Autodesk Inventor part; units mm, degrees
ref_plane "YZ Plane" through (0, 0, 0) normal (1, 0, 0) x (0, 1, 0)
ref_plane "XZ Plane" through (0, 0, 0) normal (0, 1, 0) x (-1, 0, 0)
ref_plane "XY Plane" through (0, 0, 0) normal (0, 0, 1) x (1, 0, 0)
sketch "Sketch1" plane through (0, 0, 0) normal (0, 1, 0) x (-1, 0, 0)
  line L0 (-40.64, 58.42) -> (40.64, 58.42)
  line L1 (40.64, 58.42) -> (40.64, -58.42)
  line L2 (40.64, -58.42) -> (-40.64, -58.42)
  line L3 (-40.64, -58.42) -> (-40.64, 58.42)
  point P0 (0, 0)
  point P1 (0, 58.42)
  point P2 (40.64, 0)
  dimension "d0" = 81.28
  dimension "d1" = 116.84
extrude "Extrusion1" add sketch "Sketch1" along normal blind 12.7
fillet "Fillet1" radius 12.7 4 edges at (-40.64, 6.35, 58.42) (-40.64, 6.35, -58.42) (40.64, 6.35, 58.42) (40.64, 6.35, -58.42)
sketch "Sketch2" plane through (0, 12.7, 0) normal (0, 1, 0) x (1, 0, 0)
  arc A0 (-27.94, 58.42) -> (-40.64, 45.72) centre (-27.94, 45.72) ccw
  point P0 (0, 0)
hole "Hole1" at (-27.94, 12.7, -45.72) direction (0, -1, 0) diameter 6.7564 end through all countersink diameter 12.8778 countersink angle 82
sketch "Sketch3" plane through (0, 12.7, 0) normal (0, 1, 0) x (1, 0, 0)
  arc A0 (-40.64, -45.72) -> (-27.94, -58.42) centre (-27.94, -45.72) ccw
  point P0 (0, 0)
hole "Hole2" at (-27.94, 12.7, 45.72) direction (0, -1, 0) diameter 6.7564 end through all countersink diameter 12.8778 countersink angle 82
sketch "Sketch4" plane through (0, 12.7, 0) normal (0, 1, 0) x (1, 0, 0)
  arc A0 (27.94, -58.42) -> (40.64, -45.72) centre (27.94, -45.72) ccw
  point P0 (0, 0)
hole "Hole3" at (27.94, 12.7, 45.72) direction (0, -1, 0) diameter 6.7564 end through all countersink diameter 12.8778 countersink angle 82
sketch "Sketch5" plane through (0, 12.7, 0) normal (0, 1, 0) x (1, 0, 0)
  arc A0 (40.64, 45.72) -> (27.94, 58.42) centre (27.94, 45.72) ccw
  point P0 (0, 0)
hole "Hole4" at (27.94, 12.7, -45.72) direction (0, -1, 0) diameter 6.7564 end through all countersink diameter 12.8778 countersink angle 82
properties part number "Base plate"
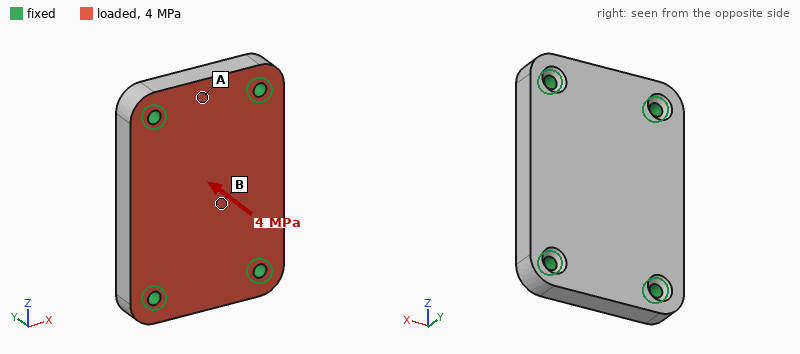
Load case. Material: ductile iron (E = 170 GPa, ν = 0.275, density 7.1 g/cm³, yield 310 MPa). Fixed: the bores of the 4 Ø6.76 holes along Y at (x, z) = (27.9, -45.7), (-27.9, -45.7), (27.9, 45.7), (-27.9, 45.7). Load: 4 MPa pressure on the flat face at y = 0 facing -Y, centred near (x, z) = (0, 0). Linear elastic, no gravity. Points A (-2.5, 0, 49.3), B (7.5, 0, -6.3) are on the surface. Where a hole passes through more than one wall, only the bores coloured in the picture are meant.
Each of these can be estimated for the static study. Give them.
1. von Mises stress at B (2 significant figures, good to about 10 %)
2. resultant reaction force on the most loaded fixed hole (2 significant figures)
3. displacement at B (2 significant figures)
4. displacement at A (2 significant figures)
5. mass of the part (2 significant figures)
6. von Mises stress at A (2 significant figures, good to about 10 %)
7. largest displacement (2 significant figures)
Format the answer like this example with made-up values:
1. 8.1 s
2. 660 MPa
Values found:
1. 50 MPa
2. 9.4 kN
3. 48 µm
4. 9.6 µm
5. 830 g
6. 30 MPa
7. 49 µm
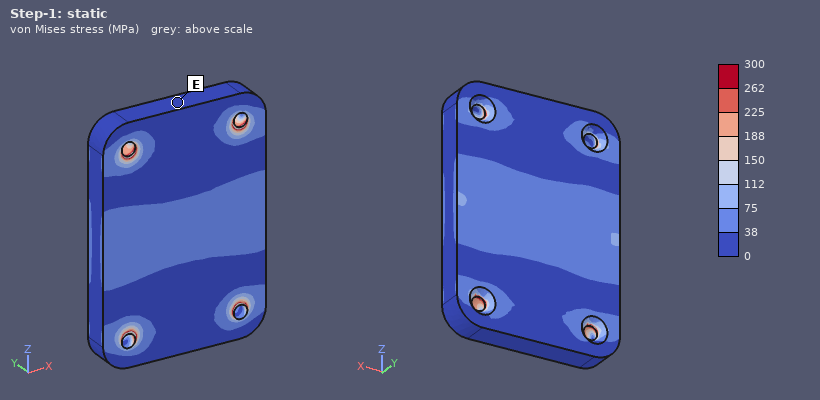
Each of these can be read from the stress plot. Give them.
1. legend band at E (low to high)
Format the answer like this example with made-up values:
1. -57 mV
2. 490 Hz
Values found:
1. 0 to 38 MPa
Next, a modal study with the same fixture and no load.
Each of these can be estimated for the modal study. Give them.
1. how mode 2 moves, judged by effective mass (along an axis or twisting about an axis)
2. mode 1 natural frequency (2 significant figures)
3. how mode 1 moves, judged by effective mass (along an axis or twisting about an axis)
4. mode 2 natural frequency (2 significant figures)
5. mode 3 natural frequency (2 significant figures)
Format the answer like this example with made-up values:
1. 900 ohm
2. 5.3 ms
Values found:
1. twisting about Z
2. 5400 Hz
3. along Y
4. 7500 Hz
5. 12 kHz
